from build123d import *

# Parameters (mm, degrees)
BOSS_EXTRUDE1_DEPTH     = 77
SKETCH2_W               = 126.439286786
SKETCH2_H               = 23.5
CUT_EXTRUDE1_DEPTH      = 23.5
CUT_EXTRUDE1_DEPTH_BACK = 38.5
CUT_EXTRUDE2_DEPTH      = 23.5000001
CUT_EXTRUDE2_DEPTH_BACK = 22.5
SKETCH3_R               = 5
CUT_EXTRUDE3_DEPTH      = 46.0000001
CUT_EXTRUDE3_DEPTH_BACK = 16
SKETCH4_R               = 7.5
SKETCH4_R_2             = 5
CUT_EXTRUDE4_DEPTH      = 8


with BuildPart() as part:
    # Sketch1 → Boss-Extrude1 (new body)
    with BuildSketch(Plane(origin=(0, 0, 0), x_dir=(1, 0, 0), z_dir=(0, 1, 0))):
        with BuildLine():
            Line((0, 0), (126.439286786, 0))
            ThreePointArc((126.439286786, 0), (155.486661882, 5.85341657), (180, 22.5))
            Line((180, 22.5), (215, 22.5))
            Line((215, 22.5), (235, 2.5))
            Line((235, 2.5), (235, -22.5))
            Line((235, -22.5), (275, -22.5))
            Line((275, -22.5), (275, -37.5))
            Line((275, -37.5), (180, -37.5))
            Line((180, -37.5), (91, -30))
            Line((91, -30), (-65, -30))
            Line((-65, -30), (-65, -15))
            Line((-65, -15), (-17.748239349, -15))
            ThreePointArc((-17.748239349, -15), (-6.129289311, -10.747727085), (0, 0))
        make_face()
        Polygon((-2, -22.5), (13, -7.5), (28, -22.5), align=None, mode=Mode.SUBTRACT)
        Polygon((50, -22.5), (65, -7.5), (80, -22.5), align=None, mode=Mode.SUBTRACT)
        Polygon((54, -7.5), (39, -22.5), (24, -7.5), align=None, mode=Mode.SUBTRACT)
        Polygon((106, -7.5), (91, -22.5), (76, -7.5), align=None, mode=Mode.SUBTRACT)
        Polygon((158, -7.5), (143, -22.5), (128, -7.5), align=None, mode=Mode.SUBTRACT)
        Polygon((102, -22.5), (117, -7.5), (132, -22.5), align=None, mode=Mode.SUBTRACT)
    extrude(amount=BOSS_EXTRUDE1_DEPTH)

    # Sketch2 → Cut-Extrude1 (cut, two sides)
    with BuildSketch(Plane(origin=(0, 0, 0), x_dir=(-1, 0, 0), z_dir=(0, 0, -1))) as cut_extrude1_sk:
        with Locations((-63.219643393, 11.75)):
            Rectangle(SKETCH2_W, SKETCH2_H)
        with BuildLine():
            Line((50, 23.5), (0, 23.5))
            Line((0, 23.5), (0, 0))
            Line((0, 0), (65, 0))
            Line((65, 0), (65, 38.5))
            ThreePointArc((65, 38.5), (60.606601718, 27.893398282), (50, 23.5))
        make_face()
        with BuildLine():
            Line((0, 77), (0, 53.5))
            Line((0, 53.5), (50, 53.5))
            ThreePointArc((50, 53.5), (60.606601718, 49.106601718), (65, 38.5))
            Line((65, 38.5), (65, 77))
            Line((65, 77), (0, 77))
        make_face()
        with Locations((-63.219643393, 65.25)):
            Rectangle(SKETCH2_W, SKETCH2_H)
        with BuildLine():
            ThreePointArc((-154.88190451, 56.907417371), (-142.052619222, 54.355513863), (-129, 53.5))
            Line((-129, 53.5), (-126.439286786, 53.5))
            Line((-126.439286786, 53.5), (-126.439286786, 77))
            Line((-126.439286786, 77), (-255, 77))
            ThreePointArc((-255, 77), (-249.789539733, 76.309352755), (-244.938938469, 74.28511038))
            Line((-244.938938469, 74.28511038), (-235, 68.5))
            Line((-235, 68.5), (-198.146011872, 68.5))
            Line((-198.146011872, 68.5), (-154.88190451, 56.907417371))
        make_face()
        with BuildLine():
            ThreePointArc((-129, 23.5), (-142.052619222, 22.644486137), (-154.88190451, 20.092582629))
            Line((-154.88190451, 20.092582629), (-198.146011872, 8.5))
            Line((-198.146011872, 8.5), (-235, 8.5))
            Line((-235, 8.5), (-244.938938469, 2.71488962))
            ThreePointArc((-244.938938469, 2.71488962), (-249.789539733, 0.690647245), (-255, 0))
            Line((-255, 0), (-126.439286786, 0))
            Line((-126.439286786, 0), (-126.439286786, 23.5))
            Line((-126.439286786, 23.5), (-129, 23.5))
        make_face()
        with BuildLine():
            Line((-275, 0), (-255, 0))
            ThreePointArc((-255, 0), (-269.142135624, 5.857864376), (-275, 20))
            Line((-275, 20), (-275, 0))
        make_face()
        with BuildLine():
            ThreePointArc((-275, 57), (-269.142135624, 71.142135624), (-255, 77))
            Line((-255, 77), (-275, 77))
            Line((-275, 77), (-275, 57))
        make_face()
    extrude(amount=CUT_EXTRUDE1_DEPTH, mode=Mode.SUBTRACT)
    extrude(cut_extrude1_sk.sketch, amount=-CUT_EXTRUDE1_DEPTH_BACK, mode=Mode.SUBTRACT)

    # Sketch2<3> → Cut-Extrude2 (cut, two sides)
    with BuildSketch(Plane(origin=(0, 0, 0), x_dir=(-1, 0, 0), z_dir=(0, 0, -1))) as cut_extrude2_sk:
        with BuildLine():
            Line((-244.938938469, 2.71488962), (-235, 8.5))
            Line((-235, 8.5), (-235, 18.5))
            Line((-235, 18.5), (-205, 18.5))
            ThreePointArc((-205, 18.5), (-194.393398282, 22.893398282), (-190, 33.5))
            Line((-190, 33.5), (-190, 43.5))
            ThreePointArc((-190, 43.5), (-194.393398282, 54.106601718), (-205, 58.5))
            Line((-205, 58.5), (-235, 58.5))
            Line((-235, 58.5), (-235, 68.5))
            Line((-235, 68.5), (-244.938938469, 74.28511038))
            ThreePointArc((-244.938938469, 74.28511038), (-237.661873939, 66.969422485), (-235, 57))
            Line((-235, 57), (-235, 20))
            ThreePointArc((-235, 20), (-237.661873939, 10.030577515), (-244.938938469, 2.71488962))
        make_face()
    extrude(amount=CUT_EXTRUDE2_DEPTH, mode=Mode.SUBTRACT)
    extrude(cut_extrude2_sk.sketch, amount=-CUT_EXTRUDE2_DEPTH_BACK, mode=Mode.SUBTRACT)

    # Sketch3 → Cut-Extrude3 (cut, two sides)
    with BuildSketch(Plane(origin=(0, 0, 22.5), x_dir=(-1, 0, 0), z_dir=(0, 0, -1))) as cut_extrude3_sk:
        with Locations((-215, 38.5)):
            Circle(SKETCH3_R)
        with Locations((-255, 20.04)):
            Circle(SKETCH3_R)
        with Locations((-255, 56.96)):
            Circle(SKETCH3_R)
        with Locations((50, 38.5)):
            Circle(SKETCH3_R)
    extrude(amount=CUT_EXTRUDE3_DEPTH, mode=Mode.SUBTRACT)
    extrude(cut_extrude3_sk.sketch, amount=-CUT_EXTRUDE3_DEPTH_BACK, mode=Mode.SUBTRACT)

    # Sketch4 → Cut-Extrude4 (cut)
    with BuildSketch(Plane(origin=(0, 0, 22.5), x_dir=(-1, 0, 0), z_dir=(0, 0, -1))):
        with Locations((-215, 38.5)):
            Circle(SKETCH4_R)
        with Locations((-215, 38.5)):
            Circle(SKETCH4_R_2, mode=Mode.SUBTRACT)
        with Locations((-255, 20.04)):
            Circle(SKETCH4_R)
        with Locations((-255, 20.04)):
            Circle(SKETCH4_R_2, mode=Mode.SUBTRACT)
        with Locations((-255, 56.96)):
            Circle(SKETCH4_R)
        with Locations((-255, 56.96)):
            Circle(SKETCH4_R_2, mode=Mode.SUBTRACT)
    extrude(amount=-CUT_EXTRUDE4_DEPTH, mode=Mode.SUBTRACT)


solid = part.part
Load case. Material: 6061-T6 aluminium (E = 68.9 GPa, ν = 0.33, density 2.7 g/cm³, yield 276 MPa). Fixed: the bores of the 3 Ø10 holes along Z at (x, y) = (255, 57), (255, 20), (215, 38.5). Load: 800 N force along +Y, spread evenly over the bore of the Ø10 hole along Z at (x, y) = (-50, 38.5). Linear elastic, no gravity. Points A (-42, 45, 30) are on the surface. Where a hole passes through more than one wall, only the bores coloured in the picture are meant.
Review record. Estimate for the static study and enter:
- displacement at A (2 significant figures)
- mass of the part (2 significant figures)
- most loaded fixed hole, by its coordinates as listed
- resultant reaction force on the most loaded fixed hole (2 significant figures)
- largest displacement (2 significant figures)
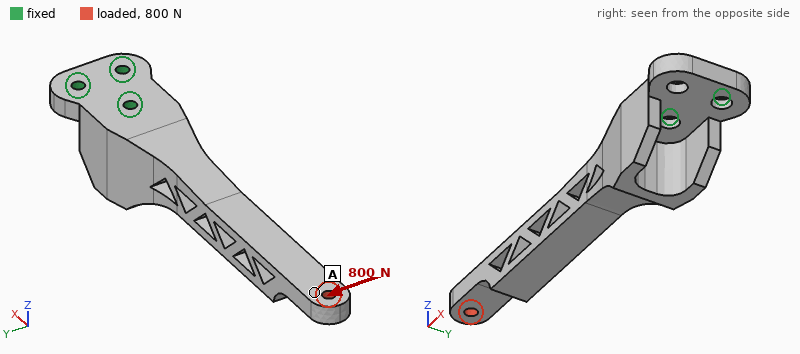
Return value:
0.92 mm
910 g
(215, 38.5)
3.4 kN
1.1 mm
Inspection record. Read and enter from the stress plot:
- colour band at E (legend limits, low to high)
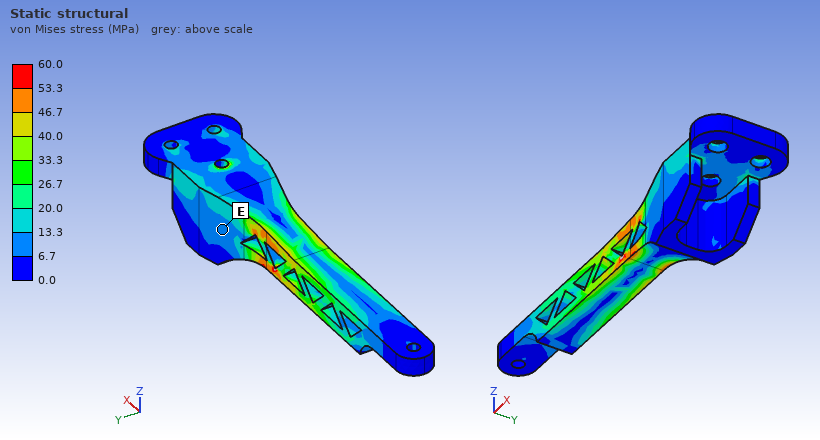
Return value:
6.7 to 13.3 MPa
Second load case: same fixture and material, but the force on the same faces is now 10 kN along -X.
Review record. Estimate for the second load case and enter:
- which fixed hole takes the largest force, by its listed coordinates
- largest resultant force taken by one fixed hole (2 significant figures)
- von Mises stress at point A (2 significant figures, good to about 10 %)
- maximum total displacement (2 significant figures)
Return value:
(215, 38.5)
5.1 kN
30 MPa
0.20 mm
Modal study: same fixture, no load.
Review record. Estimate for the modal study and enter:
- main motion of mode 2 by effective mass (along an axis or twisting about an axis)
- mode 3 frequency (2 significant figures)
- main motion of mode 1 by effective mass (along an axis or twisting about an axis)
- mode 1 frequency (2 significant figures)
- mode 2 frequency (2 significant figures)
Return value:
along Y
1700 Hz
along Z
440 Hz
480 Hz
